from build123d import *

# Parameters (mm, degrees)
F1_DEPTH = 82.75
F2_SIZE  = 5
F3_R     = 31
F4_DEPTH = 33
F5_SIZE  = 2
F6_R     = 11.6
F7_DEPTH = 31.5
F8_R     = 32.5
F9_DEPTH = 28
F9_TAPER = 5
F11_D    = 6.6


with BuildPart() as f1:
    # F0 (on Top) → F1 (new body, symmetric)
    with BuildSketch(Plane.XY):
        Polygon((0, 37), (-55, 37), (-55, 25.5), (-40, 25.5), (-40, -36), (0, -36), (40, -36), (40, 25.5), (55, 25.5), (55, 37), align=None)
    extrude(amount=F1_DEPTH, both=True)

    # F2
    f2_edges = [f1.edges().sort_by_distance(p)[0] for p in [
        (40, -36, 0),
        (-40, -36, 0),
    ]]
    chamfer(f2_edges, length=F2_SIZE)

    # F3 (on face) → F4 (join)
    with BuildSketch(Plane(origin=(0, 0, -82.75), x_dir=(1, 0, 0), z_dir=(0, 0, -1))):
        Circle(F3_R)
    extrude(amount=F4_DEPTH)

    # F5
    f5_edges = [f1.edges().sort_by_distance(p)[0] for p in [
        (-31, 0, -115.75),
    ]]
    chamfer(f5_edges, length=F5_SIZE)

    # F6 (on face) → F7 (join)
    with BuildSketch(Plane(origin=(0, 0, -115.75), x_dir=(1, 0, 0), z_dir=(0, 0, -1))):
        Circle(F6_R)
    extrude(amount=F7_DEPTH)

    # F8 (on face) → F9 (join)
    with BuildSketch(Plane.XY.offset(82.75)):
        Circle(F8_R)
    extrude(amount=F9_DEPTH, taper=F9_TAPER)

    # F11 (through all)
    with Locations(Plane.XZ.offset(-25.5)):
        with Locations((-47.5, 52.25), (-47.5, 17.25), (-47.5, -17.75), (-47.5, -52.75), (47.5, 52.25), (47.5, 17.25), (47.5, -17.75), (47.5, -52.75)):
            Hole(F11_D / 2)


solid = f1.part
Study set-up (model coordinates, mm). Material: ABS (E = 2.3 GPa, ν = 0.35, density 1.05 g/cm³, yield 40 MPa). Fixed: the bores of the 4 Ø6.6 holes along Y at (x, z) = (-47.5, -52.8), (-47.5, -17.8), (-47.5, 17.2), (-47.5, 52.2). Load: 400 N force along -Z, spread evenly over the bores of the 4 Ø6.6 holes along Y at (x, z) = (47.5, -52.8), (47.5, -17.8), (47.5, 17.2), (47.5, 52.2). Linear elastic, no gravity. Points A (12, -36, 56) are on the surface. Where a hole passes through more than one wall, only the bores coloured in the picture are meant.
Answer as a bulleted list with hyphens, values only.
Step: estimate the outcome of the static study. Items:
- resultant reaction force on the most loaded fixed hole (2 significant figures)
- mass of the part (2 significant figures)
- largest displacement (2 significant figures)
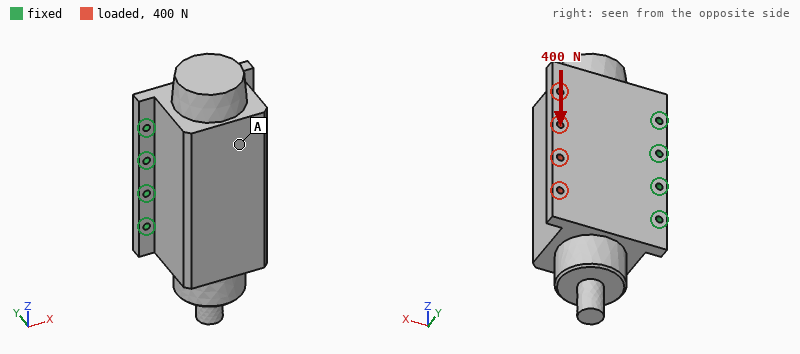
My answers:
- 330 N
- 1.3 kg
- 60 µm
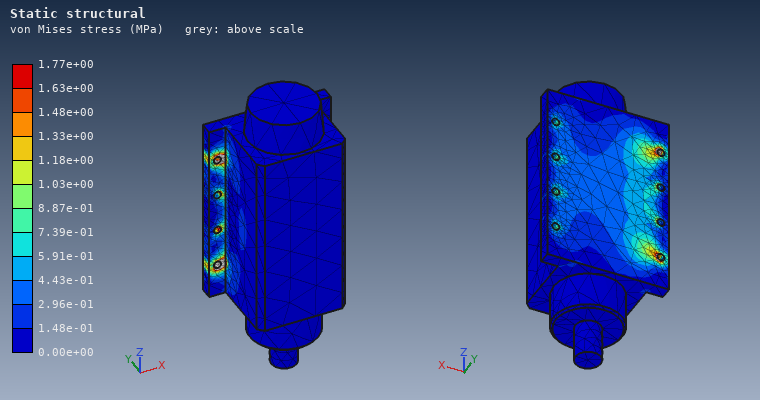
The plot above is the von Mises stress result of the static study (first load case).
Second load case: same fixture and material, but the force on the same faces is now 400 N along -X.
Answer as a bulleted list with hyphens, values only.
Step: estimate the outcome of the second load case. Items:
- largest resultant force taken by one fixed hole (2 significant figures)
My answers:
- 100 N
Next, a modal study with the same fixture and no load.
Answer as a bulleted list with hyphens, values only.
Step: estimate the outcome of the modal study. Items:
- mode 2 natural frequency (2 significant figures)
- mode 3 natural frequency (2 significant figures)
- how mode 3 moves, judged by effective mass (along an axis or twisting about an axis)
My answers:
- 480 Hz
- 620 Hz
- along Z
